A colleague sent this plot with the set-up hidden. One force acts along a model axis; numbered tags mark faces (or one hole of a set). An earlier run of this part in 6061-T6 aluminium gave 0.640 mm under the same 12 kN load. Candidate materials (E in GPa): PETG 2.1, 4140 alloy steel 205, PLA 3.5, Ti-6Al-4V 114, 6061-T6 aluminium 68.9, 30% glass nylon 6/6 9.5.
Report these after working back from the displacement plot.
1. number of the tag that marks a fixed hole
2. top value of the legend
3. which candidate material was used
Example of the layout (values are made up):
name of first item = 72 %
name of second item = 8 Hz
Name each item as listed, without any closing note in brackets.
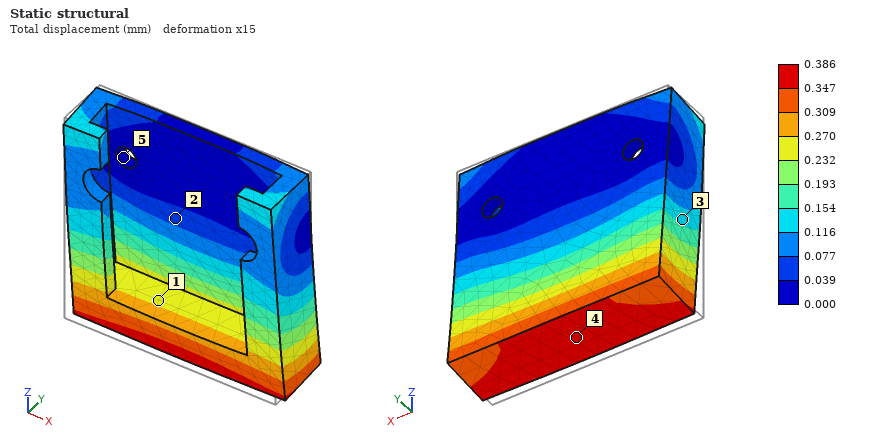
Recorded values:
number of the tag that marks a fixed hole = 5
top value of the legend = 0.386 mm
which candidate material was used = Ti-6Al-4V
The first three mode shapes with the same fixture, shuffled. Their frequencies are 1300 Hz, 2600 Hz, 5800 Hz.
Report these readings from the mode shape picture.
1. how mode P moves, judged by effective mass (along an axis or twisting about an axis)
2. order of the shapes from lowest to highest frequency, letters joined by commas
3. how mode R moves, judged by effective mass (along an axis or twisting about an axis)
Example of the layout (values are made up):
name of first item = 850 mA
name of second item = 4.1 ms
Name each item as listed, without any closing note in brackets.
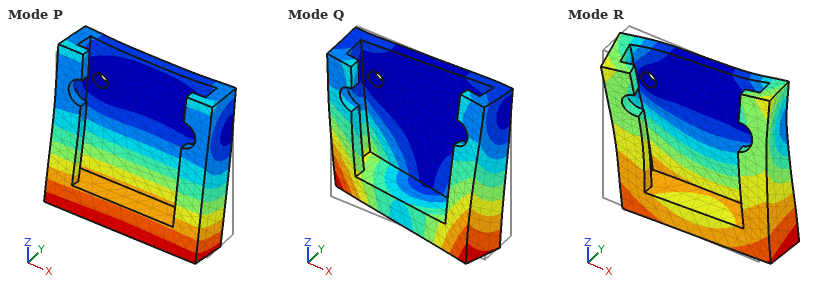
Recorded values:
how mode P moves, judged by effective mass = along Y
order of the shapes from lowest to highest frequency, letters joined by commas = P, Q, R
how mode R moves, judged by effective mass = along X
